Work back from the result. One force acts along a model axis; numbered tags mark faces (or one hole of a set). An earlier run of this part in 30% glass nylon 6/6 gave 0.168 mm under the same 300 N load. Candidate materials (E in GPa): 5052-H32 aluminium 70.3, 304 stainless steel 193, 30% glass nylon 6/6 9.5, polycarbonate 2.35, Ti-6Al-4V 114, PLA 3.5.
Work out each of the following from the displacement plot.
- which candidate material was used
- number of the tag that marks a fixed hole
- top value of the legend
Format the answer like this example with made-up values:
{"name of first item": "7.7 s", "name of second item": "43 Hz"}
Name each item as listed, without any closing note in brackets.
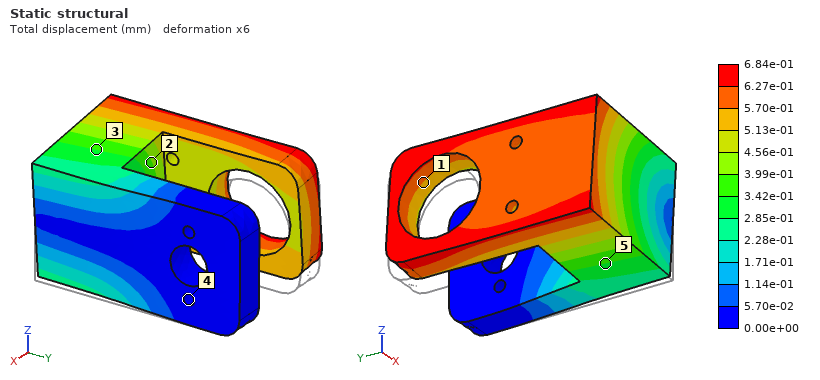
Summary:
{"which candidate material was used": "polycarbonate", "number of the tag that marks a fixed hole": "4", "top value of the legend": "6.84e-01 mm"}
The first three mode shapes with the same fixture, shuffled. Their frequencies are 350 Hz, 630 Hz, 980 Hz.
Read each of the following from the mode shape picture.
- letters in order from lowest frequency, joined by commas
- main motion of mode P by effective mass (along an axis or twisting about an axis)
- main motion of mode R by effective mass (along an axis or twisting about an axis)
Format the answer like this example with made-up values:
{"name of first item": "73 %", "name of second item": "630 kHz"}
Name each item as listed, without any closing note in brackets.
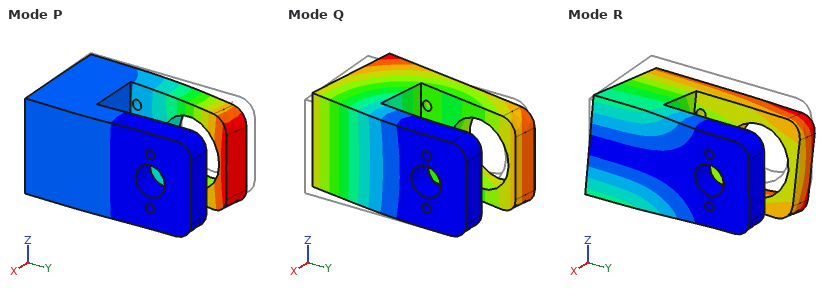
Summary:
{"letters in order from lowest frequency, joined by commas": "Q, R, P", "main motion of mode P by effective mass": "along X", "main motion of mode R by effective mass": "along Z"}
